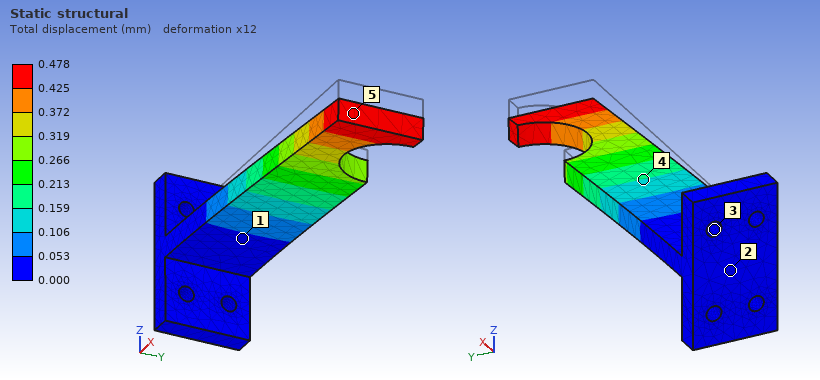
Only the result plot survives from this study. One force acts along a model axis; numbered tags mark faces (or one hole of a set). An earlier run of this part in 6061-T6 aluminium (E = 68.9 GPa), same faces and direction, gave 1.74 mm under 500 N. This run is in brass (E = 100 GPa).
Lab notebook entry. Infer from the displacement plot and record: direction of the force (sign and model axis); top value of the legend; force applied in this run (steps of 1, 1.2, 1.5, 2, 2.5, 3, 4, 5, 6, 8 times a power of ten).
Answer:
-Z
0.478 mm
200 N
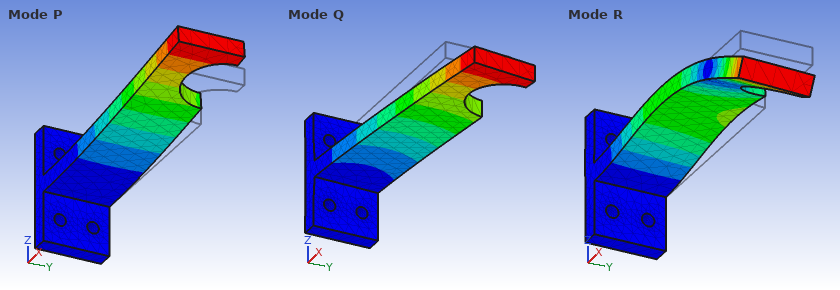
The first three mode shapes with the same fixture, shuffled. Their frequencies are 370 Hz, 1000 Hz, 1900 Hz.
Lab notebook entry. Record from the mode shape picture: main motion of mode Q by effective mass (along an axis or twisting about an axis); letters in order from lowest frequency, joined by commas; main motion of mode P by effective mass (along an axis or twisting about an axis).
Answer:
along Y
P, Q, R
along Z
